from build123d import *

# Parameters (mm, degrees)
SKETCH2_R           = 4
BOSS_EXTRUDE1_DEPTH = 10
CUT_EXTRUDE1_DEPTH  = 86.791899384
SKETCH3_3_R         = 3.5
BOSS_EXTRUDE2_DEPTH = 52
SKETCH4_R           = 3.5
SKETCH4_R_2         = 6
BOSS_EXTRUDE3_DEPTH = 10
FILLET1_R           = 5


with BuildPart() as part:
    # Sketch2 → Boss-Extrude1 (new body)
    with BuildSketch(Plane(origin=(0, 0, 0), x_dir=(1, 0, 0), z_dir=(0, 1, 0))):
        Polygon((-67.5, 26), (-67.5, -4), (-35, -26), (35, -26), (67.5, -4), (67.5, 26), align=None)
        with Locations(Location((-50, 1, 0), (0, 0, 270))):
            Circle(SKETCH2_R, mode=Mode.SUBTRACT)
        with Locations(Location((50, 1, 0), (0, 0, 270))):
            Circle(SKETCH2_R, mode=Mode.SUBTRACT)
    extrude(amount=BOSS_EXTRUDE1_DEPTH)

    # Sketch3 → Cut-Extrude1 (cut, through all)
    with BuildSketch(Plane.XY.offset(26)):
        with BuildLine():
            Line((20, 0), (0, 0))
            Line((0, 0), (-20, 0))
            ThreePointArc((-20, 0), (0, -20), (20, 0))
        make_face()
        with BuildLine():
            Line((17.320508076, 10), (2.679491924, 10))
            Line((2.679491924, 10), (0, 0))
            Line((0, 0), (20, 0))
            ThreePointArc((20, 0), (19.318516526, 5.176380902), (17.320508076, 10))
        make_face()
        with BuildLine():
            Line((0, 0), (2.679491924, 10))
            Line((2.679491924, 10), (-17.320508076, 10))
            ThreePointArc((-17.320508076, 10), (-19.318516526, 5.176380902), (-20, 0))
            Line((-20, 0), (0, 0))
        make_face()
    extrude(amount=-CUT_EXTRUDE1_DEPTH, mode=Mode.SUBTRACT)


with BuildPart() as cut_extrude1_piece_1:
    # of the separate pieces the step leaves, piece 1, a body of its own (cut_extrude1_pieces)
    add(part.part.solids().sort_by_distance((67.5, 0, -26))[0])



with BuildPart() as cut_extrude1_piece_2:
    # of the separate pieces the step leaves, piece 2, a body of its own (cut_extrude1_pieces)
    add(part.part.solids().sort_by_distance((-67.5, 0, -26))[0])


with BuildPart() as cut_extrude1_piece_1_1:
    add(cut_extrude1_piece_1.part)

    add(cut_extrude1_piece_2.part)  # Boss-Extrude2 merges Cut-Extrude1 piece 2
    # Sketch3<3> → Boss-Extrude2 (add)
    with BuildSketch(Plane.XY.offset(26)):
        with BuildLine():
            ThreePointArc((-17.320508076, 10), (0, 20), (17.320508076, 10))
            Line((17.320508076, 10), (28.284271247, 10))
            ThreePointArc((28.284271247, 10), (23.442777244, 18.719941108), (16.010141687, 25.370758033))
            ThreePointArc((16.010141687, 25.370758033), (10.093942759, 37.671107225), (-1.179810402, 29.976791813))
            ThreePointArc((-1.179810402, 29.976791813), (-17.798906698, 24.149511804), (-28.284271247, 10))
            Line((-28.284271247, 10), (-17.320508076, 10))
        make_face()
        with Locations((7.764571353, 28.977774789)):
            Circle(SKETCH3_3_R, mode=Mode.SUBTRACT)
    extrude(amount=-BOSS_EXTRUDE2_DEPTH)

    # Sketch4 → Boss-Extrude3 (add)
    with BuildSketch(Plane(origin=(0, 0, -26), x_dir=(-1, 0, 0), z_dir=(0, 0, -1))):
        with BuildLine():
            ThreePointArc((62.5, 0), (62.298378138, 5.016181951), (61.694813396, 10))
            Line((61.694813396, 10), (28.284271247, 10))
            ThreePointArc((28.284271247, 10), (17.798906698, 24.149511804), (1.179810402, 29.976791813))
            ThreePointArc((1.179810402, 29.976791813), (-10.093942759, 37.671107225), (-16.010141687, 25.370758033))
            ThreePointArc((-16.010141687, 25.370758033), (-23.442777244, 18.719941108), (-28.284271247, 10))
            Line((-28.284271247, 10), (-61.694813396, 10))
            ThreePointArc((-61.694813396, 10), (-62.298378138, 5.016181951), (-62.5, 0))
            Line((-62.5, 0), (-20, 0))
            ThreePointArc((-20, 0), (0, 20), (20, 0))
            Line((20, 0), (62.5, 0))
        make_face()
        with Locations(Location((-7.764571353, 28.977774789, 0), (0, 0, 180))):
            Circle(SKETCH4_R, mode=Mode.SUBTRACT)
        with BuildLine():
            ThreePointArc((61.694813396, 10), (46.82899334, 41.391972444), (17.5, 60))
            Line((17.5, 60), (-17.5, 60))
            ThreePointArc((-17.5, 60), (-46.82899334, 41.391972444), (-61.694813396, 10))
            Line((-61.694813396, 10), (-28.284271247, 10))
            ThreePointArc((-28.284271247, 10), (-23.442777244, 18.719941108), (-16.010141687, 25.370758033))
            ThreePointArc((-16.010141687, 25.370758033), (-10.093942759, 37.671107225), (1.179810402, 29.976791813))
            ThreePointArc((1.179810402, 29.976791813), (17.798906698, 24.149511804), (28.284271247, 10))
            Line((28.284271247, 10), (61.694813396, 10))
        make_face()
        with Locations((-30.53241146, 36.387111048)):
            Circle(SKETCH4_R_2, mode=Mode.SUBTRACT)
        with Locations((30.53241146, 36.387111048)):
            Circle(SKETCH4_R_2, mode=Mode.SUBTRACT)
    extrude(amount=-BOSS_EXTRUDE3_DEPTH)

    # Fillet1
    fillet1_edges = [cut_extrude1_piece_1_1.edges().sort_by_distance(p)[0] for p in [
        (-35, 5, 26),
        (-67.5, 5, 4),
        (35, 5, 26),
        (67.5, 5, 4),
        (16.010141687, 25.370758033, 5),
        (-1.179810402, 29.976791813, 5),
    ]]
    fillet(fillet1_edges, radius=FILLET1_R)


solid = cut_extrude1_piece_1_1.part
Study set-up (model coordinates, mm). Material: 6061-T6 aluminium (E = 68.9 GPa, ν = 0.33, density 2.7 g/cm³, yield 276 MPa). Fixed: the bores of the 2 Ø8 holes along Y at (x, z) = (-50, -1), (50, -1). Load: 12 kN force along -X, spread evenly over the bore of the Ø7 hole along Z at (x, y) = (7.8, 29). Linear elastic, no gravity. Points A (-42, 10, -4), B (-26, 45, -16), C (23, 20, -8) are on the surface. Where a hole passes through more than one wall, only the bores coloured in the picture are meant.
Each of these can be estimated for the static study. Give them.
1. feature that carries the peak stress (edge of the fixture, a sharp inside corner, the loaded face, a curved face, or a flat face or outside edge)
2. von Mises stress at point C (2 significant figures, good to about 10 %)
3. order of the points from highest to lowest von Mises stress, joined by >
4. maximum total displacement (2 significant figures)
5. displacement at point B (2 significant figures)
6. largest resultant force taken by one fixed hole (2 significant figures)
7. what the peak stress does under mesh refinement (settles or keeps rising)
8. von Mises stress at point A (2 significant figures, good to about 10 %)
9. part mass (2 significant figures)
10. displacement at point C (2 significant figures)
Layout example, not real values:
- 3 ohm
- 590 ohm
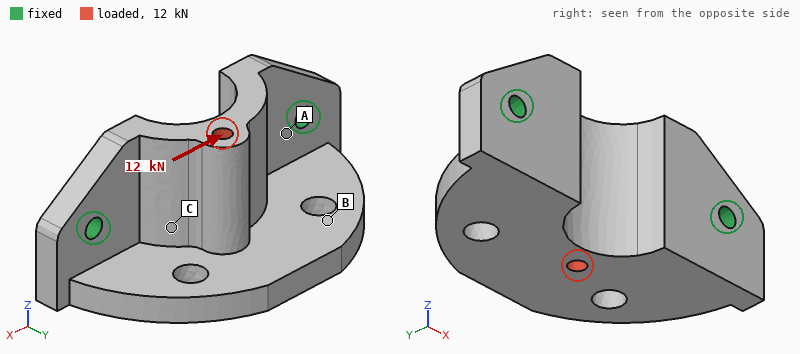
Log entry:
- edge of the fixture
- 17 MPa
- A > C > B
- 38 µm
- 24 µm
- 6.9 kN
- keeps rising
- 31 MPa
- 310 g
- 20 µm
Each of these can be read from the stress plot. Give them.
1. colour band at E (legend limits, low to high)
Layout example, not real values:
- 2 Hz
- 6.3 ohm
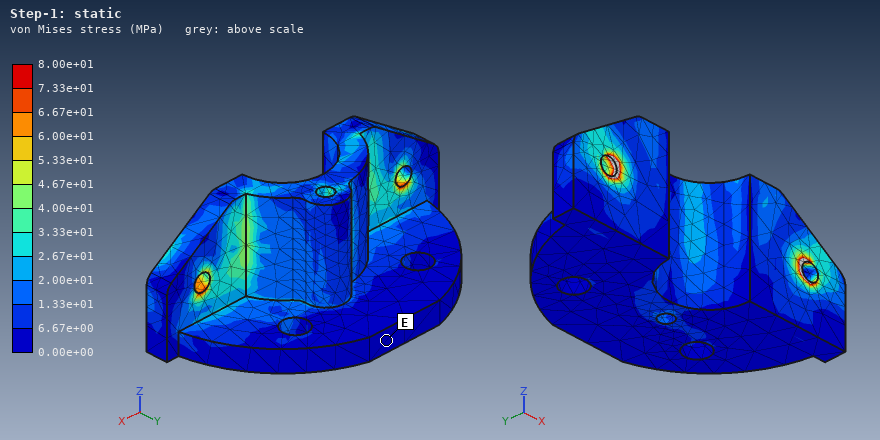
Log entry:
- 0.00e+00 to 6.67e+00 MPa
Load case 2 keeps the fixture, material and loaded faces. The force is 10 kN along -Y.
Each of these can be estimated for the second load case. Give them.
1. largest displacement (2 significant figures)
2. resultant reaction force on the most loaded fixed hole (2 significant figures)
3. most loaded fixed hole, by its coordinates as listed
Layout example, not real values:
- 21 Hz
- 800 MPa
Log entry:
- 0.10 mm
- 8.1 kN
- (50, -1)
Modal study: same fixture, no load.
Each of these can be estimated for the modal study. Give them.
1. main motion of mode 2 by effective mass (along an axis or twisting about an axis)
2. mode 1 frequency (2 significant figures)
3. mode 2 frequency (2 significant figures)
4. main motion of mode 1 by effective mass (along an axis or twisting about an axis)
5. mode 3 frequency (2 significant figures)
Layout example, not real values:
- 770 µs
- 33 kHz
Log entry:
- along Y
- 2100 Hz
- 5400 Hz
- along Z
- 5700 Hz
